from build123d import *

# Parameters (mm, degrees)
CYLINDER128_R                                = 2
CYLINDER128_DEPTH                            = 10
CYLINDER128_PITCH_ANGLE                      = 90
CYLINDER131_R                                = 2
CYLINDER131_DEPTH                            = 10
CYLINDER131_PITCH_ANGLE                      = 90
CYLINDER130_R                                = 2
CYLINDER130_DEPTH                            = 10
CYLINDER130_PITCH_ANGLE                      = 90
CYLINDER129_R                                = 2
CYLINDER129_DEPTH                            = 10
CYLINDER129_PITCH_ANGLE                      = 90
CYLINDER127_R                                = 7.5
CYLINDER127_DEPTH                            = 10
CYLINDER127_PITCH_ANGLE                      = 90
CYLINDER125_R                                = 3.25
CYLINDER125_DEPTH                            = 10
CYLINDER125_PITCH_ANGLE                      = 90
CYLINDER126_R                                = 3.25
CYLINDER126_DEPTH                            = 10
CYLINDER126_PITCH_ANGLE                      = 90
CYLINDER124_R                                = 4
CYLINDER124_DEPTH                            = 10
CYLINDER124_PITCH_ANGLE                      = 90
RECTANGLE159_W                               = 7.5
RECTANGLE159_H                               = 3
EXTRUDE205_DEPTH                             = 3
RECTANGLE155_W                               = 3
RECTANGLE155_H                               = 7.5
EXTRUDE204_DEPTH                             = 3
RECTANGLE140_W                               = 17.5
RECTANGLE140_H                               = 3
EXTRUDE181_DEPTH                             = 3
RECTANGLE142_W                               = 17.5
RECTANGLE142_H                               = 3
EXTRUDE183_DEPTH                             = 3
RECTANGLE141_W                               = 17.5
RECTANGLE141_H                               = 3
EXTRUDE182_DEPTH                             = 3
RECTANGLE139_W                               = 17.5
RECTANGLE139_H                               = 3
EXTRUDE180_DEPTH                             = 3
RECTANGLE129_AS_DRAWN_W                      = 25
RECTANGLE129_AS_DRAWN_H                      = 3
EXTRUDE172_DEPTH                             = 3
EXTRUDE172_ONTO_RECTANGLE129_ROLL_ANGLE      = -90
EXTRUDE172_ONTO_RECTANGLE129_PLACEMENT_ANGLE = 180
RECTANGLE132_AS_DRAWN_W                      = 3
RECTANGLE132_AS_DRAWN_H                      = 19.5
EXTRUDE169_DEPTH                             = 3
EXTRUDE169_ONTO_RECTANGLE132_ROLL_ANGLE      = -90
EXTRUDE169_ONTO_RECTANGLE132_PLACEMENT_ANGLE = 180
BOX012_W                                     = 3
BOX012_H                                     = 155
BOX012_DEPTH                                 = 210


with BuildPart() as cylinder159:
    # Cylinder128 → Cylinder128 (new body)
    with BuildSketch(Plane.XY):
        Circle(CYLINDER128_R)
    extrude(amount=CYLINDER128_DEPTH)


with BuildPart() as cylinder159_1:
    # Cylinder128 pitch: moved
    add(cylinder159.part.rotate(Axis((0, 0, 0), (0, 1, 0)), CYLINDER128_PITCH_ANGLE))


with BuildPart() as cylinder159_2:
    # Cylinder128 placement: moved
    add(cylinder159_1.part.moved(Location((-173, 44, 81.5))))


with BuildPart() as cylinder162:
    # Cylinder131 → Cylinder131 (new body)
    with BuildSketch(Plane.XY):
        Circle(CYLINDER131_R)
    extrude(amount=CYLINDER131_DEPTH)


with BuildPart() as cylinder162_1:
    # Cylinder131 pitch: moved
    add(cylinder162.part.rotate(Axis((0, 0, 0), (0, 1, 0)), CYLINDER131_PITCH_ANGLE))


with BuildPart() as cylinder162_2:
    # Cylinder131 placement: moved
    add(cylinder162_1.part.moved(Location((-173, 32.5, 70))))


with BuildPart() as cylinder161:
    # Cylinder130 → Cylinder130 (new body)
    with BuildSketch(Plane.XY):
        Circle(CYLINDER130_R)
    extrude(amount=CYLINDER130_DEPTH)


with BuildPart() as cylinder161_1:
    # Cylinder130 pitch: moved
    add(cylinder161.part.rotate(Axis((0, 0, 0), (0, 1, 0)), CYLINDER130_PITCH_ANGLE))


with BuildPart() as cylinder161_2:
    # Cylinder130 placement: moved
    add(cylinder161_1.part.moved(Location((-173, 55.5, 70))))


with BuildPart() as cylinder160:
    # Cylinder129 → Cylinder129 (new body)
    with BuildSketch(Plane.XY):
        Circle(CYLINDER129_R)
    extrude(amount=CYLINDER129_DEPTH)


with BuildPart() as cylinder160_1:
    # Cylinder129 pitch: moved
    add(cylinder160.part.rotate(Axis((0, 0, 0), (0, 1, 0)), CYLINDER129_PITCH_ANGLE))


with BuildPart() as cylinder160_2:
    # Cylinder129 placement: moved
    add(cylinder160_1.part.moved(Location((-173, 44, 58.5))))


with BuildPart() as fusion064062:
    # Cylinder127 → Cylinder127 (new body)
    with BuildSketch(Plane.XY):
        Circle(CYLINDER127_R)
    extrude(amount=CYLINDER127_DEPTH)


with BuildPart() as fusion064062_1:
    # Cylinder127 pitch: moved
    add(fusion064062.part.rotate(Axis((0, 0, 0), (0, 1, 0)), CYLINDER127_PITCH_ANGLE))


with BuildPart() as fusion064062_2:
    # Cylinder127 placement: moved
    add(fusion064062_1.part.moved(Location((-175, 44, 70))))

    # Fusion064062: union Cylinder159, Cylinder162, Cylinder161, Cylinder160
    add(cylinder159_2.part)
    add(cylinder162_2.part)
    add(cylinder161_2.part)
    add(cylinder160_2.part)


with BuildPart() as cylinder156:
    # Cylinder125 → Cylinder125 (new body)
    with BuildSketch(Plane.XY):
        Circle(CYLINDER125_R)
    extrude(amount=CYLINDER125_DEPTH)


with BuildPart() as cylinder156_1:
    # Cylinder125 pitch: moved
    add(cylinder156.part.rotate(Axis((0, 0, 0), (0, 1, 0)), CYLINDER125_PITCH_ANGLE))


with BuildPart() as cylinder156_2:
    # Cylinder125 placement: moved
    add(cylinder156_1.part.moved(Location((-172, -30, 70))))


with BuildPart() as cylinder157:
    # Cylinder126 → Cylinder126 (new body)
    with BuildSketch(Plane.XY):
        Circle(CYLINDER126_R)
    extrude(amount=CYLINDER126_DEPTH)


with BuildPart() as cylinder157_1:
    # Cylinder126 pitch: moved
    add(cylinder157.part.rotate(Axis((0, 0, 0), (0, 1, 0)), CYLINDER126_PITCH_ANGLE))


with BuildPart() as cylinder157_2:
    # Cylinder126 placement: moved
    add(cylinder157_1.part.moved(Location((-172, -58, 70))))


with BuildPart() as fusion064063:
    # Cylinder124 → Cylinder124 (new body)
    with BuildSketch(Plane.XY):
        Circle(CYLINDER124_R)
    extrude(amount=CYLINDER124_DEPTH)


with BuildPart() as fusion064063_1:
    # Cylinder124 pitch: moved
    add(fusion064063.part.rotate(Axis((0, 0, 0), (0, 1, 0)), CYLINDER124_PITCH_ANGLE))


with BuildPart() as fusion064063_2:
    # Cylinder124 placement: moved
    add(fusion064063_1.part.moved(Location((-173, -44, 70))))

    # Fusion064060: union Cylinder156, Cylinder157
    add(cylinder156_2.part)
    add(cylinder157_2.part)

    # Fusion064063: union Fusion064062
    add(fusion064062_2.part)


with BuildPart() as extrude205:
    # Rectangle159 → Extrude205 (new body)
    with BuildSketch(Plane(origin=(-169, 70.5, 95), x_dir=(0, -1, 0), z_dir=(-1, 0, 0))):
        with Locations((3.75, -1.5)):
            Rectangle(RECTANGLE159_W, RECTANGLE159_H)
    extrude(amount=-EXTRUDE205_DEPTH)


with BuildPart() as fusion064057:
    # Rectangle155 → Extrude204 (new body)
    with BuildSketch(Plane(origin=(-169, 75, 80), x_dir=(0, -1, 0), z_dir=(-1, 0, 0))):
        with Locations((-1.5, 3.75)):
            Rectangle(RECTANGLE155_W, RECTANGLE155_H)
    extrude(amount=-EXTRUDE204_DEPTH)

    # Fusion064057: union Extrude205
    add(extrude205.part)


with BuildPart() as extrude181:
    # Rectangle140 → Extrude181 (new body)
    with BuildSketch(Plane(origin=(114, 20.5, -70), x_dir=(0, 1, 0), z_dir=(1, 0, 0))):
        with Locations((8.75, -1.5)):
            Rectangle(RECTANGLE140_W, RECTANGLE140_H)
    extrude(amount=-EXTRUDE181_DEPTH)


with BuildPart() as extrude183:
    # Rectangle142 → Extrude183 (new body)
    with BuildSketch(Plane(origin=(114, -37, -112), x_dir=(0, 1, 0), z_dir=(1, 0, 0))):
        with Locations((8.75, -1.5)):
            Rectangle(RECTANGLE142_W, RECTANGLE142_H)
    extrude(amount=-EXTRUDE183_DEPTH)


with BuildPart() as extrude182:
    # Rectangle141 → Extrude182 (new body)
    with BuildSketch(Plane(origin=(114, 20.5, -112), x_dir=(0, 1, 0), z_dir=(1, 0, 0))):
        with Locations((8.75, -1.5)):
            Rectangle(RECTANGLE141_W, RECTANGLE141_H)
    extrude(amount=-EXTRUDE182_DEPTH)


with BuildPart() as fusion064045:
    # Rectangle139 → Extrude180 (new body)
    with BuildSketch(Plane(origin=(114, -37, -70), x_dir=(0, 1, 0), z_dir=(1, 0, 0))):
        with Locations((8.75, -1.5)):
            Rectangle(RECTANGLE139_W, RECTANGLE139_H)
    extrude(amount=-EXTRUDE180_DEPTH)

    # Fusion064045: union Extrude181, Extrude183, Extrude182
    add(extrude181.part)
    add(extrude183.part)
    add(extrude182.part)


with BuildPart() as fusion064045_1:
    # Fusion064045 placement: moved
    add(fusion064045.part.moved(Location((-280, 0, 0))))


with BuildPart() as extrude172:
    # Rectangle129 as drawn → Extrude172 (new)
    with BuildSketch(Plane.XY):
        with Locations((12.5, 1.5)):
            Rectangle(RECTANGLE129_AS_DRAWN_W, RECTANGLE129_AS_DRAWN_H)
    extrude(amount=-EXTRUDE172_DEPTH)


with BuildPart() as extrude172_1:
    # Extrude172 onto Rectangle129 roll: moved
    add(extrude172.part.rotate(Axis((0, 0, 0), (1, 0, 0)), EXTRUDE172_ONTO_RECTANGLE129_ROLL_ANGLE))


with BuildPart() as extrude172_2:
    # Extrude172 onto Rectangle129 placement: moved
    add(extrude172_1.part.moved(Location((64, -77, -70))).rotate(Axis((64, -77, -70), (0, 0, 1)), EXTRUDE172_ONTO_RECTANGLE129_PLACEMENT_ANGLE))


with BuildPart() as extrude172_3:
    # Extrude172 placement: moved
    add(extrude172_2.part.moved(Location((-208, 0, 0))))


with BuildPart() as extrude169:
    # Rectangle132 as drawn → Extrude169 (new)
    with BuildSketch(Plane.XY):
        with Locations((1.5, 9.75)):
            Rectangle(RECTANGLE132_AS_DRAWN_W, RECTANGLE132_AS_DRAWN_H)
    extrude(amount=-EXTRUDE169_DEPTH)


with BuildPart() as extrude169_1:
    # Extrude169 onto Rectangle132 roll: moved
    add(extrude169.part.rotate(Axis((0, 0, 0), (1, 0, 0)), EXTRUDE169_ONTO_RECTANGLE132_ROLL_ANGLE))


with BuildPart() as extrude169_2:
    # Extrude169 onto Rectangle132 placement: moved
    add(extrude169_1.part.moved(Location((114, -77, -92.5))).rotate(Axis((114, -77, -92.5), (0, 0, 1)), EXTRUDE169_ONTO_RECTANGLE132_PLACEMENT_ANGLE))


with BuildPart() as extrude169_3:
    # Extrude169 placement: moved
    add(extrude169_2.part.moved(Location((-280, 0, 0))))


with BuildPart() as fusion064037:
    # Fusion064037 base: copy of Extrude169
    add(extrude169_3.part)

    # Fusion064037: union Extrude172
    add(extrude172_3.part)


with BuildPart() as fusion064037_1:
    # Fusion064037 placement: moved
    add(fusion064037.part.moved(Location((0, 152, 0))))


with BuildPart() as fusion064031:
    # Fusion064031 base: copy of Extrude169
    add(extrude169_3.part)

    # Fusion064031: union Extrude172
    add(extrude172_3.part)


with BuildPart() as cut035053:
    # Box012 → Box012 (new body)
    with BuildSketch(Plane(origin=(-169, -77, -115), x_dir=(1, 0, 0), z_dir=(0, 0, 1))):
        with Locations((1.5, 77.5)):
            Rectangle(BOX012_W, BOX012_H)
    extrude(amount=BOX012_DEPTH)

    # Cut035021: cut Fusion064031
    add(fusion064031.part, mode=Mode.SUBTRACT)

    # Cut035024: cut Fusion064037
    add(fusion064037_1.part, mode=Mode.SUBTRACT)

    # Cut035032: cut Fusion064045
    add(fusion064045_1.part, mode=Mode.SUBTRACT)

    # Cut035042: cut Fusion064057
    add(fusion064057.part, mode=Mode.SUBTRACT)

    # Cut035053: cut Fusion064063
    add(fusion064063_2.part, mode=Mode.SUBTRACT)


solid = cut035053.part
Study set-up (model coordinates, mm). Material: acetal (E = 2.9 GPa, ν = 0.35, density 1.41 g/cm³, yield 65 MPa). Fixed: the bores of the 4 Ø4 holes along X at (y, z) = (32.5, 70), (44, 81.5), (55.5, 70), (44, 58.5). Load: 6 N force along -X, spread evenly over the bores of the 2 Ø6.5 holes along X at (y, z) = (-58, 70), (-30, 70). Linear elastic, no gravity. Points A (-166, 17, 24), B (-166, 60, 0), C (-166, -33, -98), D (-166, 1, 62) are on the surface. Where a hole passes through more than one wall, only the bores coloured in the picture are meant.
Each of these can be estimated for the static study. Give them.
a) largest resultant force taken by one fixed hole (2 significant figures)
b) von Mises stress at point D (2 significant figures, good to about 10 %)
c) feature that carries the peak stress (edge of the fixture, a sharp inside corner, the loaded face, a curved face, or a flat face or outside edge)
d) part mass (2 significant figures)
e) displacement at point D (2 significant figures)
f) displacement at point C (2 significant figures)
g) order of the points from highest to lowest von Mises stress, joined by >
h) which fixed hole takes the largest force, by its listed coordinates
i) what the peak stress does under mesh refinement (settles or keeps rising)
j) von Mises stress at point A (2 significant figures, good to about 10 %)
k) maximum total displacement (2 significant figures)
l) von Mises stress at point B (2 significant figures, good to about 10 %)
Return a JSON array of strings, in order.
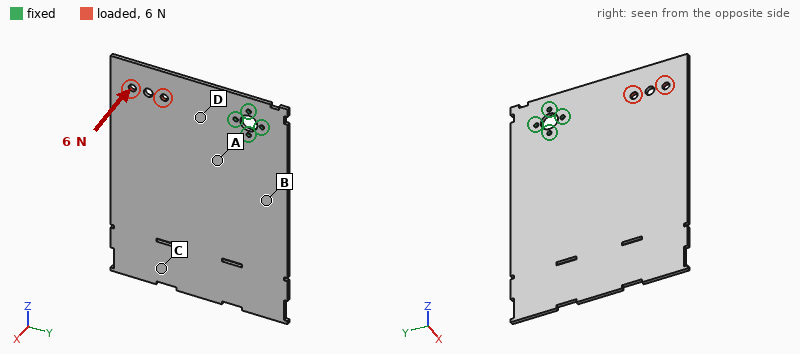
["20 N", "1.7 MPa", "edge of the fixture", "130 g", "0.46 mm", "0.69 mm", "D > A > B > C", "(32.5, 70)", "keeps rising", "1.3 MPa", "2.8 mm", "0.65 MPa"]
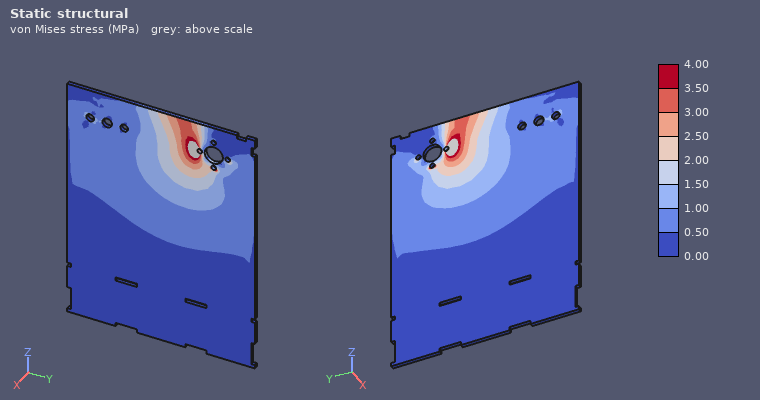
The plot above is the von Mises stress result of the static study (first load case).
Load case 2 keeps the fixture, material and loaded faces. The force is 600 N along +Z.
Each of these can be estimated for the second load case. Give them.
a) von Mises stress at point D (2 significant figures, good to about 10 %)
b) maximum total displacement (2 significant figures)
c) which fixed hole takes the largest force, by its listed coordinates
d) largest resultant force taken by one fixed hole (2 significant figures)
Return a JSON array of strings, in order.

["6.4 MPa", "2.8 mm", "(32.5, 70)", "1.3 kN"]
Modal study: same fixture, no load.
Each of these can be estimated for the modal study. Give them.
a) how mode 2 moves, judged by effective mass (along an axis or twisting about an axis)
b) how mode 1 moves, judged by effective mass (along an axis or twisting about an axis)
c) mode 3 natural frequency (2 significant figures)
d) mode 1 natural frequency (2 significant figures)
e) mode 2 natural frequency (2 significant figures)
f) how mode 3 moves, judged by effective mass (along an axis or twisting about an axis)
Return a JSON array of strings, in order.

["twisting about Z", "along X", "83 Hz", "18 Hz", "39 Hz", "along X"]
